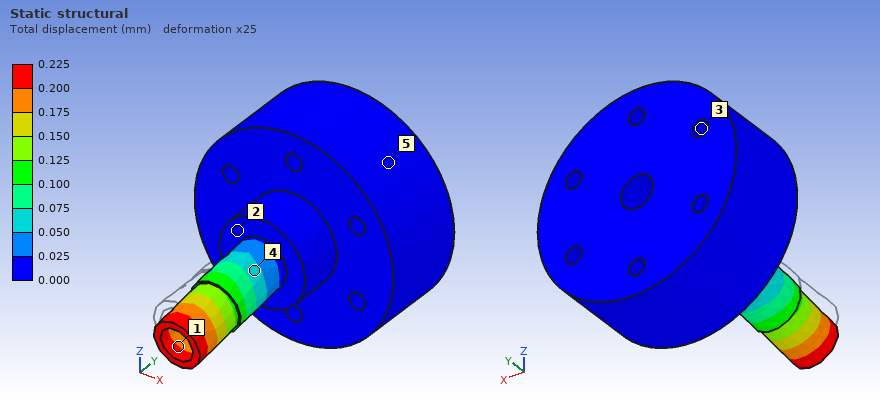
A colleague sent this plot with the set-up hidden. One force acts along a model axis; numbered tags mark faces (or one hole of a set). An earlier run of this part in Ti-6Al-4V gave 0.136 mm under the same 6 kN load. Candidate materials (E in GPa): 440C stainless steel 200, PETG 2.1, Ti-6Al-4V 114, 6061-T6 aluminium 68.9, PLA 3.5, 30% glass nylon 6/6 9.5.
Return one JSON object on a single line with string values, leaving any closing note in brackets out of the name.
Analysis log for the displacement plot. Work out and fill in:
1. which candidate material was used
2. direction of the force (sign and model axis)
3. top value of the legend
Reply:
{"which candidate material was used": "6061-T6 aluminium", "direction of the force": "-Z", "top value of the legend": "0.225 mm"}
